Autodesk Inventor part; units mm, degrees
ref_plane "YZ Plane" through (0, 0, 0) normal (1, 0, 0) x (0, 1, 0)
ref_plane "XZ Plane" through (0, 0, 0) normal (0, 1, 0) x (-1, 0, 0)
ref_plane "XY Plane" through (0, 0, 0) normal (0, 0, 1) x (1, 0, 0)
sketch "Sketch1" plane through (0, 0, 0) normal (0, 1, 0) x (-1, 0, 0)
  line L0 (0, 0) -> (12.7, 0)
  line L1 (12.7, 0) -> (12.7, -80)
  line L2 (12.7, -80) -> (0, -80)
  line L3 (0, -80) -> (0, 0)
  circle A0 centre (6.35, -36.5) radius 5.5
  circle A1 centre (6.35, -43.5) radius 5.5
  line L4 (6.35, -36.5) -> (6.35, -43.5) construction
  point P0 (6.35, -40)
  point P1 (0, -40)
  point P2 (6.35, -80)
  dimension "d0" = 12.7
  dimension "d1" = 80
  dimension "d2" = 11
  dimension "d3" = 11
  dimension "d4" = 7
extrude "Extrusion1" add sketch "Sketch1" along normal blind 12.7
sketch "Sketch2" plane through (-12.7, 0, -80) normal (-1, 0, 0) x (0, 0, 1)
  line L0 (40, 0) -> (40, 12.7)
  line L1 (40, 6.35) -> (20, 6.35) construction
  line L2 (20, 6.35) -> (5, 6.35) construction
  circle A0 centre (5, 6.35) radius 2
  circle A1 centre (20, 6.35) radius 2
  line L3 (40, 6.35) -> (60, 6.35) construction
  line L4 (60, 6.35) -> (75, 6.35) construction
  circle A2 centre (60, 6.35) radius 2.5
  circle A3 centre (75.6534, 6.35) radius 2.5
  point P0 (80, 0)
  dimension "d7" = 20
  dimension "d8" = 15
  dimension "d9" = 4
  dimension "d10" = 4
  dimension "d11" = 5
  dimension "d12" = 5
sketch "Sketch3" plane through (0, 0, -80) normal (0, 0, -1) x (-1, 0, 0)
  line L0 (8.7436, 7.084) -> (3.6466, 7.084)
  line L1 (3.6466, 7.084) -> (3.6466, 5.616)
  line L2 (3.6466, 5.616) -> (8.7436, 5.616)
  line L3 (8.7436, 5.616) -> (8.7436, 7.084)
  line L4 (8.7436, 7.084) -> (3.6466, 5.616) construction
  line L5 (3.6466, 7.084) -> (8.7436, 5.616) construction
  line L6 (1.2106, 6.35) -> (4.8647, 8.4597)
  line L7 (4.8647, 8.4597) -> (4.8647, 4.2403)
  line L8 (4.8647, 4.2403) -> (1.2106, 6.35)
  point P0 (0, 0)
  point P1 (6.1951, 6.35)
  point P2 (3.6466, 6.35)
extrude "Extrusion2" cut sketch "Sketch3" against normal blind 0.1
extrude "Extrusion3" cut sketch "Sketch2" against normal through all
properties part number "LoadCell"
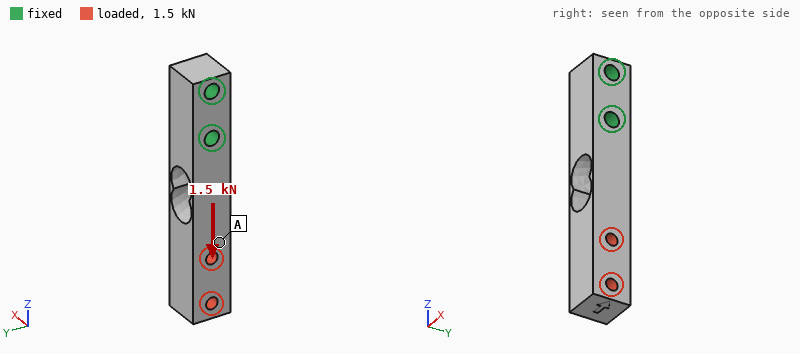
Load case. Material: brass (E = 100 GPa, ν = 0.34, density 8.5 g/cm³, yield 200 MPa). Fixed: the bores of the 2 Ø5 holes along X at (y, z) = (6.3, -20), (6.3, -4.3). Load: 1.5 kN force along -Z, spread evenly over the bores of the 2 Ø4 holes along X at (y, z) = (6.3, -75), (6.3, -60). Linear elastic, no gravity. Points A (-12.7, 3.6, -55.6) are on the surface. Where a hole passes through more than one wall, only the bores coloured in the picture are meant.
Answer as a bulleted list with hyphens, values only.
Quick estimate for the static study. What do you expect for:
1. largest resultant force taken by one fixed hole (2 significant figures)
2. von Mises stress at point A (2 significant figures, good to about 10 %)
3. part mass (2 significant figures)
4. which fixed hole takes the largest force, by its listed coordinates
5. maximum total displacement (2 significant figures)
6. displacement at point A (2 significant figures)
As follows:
- 1.4 kN
- 15 MPa
- 85 g
- (6.3, -20)
- 15 µm
- 13 µm
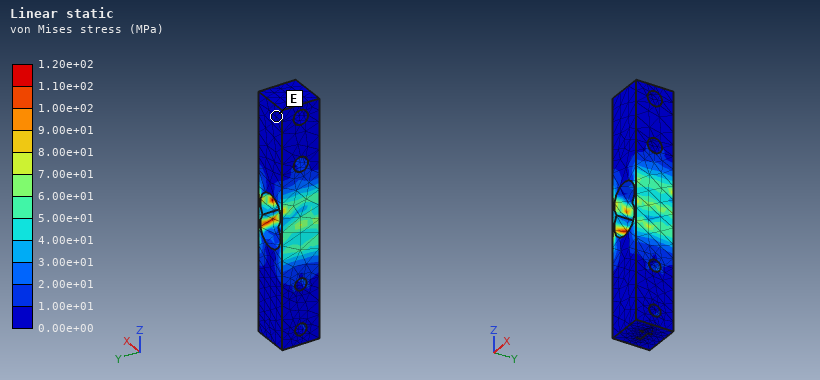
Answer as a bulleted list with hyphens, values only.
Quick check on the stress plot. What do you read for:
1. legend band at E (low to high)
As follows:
- 0.00e+00 to 1.00e+01 MPa
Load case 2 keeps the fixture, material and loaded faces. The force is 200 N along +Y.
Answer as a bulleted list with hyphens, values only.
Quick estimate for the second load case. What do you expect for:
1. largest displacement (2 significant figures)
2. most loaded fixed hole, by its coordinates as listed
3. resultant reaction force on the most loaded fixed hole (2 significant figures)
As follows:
- 0.16 mm
- (6.3, -20)
- 410 N
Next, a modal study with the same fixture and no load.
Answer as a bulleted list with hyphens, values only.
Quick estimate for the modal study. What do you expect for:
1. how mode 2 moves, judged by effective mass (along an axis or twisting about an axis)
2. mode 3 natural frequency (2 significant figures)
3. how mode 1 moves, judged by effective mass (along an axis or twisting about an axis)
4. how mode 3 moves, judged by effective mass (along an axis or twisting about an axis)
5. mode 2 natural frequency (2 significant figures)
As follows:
- along Y
- 4200 Hz
- along X
- twisting about Z
- 1100 Hz
